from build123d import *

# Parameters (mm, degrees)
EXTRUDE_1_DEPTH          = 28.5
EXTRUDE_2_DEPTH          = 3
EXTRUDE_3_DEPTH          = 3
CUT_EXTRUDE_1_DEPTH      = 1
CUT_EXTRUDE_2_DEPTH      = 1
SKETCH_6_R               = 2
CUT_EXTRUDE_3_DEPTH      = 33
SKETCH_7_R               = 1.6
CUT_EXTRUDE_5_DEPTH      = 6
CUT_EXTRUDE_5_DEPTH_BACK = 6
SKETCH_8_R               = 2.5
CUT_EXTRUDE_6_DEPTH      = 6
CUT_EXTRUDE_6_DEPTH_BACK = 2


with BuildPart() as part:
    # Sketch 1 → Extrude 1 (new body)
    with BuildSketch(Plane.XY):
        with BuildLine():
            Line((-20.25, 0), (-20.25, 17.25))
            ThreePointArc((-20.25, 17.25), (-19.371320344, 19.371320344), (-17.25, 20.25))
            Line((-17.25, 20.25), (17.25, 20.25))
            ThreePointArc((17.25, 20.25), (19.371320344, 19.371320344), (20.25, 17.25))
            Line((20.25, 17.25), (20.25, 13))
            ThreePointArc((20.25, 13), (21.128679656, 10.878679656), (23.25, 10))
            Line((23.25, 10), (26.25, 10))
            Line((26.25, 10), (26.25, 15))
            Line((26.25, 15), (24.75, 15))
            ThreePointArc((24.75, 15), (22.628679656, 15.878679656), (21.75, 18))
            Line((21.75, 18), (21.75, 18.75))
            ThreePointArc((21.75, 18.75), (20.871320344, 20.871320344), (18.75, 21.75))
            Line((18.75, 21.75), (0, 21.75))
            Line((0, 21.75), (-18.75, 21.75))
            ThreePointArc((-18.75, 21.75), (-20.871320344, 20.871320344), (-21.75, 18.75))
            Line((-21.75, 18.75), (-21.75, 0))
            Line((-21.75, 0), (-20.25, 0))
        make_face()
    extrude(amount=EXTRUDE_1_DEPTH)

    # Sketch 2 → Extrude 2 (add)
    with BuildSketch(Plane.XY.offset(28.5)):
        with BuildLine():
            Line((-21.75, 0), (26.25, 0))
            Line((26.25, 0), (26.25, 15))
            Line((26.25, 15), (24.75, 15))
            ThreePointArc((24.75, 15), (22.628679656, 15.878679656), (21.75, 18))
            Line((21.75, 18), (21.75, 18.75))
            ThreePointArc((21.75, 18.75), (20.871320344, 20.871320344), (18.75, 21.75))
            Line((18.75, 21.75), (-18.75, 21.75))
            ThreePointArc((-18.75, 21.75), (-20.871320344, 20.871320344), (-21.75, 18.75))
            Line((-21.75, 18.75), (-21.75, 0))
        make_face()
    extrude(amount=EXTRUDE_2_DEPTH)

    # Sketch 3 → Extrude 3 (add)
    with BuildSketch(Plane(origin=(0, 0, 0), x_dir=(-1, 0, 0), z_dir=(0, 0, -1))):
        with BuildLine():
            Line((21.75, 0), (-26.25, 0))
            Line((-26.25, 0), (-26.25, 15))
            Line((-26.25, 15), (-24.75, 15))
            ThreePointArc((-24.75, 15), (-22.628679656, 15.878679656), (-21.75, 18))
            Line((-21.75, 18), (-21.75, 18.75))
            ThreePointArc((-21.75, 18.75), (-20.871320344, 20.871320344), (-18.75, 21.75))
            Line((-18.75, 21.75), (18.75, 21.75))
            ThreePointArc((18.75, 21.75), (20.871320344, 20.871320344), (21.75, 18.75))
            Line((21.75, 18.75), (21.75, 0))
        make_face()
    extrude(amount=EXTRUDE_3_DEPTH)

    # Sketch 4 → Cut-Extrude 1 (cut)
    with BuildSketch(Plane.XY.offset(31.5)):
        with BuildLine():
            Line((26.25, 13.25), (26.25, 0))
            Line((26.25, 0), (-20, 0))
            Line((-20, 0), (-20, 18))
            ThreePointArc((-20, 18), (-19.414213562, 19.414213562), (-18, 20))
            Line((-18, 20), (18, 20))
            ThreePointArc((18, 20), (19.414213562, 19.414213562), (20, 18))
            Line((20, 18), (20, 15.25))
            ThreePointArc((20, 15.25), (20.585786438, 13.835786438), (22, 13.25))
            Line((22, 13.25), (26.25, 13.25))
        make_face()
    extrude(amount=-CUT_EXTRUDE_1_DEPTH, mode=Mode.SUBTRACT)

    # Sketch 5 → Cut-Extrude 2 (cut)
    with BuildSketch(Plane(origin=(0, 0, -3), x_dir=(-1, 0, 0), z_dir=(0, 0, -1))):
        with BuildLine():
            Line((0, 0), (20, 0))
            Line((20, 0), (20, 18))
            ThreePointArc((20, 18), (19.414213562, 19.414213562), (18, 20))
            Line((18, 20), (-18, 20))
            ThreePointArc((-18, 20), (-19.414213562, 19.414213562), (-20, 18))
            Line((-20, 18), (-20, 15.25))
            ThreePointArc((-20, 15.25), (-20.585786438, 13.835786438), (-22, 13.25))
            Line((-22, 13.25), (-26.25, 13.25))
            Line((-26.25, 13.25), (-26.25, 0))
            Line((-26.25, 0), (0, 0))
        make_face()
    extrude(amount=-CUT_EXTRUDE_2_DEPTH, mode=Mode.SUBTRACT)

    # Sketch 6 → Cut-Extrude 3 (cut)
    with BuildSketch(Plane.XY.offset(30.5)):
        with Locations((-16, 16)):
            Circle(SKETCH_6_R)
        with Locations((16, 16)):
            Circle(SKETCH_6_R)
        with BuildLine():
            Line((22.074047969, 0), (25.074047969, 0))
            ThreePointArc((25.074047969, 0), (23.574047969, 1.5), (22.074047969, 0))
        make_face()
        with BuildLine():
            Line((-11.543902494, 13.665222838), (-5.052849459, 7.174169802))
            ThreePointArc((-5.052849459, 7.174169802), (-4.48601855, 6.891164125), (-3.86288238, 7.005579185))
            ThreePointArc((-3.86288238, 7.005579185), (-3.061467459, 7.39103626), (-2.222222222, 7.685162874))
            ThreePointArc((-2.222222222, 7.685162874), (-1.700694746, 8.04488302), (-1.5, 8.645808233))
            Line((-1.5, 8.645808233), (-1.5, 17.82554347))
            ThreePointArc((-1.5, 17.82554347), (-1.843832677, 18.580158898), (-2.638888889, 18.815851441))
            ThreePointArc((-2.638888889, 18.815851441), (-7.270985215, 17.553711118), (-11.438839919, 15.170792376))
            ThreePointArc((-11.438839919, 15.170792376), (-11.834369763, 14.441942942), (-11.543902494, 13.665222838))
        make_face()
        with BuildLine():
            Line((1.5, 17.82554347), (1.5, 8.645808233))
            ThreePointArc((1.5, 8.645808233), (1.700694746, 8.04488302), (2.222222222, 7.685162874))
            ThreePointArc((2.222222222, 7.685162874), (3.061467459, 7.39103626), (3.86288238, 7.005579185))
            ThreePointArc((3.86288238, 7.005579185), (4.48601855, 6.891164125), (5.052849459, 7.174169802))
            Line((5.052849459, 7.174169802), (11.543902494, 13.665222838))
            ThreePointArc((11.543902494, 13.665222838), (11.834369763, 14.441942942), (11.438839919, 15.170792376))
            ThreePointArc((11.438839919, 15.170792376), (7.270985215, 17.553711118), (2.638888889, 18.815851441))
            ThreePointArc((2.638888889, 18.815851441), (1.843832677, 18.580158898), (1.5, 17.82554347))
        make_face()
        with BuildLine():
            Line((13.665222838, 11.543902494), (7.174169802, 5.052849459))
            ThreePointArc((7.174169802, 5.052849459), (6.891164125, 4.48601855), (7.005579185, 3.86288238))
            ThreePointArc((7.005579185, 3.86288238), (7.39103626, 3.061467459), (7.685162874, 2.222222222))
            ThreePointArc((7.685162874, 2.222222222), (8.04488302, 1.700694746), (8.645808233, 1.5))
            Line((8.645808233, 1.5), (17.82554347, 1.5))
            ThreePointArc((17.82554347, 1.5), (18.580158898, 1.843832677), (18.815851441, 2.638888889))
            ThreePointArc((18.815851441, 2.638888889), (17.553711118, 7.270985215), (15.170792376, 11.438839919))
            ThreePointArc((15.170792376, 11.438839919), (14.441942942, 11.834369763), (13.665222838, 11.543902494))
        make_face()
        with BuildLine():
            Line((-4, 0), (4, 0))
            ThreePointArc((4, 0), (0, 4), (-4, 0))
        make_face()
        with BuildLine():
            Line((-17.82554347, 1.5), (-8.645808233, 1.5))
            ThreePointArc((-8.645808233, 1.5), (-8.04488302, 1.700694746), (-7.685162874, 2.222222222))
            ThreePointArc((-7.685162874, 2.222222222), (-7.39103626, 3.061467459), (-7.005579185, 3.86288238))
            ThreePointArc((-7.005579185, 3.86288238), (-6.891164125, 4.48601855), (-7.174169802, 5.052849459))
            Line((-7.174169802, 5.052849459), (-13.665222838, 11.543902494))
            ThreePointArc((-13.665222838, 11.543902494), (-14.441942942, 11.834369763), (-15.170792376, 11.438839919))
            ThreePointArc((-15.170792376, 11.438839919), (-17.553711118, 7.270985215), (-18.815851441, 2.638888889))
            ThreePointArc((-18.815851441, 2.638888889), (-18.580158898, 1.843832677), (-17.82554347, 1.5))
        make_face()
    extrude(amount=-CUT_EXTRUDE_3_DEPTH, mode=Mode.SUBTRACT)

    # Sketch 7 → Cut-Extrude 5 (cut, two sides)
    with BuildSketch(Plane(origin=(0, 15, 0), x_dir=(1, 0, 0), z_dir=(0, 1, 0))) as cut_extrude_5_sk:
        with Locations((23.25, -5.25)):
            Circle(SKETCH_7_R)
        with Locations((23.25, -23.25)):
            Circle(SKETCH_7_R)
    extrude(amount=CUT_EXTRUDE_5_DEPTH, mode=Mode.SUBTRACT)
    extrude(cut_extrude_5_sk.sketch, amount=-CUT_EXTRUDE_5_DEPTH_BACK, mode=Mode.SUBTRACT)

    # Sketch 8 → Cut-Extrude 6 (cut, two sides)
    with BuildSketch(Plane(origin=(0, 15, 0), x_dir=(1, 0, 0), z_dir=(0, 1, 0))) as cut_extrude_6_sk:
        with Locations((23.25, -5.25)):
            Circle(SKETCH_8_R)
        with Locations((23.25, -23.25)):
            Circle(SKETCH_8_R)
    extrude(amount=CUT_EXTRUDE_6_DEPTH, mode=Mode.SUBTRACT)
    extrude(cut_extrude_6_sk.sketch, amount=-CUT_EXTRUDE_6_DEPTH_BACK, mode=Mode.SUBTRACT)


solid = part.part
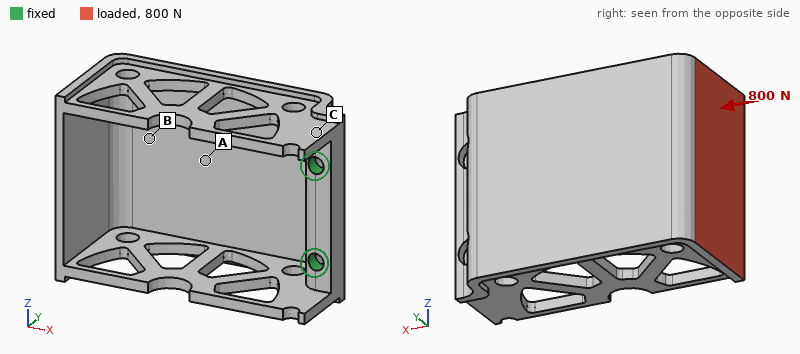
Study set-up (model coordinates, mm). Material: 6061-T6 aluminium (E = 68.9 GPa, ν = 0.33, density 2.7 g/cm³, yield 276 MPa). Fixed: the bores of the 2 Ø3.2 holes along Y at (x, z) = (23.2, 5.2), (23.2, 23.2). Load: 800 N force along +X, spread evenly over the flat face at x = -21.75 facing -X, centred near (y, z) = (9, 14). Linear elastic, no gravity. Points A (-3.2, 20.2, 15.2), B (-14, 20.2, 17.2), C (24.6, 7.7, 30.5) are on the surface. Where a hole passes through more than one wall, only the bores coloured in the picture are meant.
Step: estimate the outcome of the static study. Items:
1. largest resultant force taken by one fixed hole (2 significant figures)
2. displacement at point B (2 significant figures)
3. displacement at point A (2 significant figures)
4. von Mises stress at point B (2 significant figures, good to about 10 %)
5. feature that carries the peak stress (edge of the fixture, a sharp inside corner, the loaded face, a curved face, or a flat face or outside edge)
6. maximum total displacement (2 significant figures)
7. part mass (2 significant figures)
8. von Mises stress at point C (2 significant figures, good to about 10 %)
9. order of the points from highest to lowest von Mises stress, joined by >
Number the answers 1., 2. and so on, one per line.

1. 400 N
2. 0.12 mm
3. 0.076 mm
4. 46 MPa
5. a curved face
6. 0.39 mm
7. 17 g
8. 30 MPa
9. B > C > A
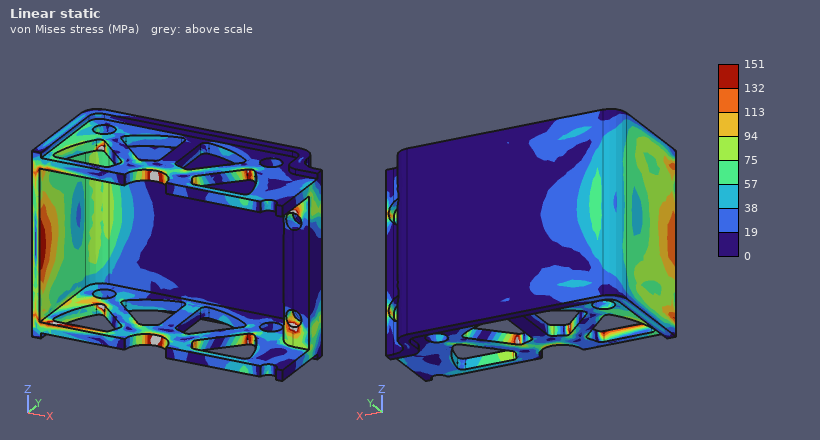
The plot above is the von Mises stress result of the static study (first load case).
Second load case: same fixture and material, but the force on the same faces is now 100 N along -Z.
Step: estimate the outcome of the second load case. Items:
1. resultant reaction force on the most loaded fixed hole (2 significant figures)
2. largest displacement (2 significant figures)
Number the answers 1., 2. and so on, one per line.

1. 170 N
2. 0.34 mm
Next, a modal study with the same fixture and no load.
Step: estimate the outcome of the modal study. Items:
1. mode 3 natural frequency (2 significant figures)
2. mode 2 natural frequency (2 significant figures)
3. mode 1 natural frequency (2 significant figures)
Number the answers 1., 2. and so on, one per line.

1. 5000 Hz
2. 1300 Hz
3. 1300 Hz
